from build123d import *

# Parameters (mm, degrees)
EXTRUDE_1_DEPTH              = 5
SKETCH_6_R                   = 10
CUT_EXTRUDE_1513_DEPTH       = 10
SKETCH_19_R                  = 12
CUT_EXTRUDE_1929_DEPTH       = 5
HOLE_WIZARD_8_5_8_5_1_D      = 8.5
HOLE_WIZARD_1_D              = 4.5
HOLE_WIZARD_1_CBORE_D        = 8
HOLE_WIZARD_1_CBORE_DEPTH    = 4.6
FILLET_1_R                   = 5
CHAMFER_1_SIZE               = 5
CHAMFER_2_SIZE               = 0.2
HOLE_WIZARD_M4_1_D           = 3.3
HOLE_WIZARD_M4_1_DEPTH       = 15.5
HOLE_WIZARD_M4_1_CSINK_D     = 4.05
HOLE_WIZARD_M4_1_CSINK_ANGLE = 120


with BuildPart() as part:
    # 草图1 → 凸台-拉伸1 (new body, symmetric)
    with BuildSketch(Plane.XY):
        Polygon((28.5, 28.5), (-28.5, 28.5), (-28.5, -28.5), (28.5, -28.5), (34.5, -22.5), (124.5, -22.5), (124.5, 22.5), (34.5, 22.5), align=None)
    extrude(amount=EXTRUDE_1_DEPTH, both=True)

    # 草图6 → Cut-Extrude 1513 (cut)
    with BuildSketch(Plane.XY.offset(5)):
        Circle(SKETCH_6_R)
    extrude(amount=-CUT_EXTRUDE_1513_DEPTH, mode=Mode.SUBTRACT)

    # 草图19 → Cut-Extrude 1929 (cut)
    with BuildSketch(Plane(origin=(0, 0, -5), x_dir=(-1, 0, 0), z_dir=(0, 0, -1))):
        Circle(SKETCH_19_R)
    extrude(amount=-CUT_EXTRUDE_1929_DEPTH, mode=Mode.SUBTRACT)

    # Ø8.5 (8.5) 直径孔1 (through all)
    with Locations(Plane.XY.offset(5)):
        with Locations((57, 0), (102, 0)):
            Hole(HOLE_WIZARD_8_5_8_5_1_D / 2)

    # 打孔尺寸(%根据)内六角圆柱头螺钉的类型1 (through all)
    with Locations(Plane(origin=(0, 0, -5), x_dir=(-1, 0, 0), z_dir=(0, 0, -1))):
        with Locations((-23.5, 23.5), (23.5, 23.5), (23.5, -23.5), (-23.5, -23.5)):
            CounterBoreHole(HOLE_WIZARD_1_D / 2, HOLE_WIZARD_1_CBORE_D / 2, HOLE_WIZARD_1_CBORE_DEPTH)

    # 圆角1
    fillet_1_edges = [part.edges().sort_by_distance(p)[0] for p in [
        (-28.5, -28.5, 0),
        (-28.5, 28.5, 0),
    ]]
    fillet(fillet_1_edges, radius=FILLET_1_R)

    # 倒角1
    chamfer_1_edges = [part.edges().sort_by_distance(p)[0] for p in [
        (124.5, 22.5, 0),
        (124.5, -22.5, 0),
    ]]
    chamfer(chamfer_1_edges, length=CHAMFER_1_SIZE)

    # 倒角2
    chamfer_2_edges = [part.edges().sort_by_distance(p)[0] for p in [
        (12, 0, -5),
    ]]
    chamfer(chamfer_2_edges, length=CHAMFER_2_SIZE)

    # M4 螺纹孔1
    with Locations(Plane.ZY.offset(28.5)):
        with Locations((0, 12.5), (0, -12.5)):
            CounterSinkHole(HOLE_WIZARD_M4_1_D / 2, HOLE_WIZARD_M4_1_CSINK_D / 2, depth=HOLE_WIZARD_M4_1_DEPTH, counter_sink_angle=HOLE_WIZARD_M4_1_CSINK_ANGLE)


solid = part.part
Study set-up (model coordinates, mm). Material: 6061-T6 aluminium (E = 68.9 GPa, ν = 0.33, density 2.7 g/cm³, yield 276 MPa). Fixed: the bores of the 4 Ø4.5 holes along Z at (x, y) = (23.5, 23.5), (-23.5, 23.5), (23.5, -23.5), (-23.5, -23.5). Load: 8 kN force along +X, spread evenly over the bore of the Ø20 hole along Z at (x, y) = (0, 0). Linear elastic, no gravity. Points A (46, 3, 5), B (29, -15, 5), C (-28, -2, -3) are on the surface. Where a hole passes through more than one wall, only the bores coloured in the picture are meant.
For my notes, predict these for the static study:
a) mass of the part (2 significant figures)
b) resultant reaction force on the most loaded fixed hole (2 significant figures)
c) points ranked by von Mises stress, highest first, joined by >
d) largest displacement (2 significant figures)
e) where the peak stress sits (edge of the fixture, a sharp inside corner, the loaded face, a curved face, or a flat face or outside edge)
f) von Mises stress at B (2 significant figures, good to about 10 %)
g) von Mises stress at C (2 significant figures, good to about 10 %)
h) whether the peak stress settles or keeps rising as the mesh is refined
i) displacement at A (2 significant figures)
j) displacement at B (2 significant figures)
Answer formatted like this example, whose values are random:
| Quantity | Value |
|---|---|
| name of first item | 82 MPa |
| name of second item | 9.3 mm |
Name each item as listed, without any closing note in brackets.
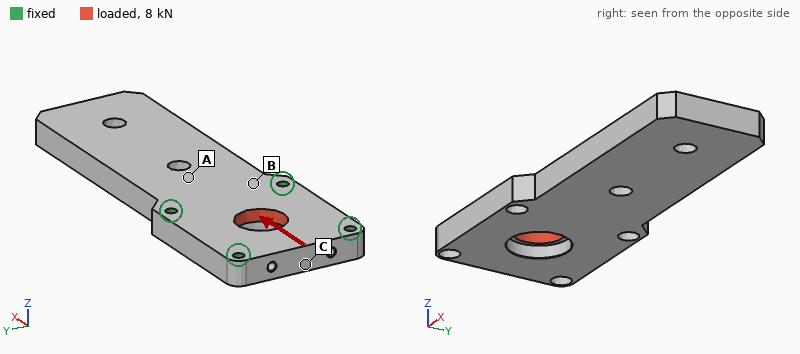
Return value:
| Quantity | Value |
|---|---|
| mass of the part | 190 g |
| resultant reaction force on the most loaded fixed hole | 2.3 kN |
| points ranked by von Mises stress, highest first, joined by > | C > B > A |
| largest displacement | 13 µm |
| where the peak stress sits | edge of the fixture |
| von Mises stress at B | 8.0 MPa |
| von Mises stress at C | 17 MPa |
| whether the peak stress settles or keeps rising as the mesh is refined | keeps rising |
| displacement at A | 3.6 µm |
| displacement at B | 2.8 µm |
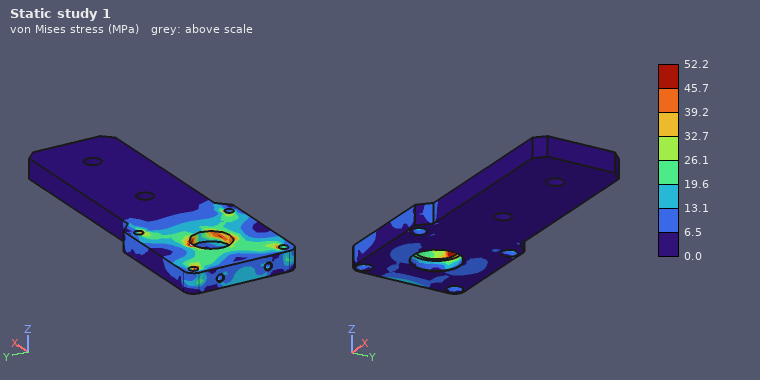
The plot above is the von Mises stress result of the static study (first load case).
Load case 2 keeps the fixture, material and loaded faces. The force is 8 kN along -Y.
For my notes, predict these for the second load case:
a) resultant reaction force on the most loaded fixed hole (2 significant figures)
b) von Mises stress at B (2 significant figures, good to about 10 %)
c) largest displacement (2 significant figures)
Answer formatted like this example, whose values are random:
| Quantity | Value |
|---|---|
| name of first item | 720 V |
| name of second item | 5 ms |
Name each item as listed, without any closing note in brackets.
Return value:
| Quantity | Value |
|---|---|
| resultant reaction force on the most loaded fixed hole | 2.2 kN |
| von Mises stress at B | 7.9 MPa |
| largest displacement | 13 µm |
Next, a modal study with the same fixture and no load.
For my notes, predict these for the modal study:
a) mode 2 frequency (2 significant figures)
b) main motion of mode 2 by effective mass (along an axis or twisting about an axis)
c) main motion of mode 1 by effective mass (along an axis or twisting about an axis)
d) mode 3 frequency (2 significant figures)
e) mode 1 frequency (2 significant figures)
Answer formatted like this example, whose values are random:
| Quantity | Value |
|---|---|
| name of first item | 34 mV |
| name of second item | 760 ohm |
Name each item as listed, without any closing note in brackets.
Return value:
| Quantity | Value |
|---|---|
| mode 2 frequency | 3100 Hz |
| main motion of mode 2 by effective mass | along Y |
| main motion of mode 1 by effective mass | along Z |
| mode 3 frequency | 3400 Hz |
| mode 1 frequency | 690 Hz |
